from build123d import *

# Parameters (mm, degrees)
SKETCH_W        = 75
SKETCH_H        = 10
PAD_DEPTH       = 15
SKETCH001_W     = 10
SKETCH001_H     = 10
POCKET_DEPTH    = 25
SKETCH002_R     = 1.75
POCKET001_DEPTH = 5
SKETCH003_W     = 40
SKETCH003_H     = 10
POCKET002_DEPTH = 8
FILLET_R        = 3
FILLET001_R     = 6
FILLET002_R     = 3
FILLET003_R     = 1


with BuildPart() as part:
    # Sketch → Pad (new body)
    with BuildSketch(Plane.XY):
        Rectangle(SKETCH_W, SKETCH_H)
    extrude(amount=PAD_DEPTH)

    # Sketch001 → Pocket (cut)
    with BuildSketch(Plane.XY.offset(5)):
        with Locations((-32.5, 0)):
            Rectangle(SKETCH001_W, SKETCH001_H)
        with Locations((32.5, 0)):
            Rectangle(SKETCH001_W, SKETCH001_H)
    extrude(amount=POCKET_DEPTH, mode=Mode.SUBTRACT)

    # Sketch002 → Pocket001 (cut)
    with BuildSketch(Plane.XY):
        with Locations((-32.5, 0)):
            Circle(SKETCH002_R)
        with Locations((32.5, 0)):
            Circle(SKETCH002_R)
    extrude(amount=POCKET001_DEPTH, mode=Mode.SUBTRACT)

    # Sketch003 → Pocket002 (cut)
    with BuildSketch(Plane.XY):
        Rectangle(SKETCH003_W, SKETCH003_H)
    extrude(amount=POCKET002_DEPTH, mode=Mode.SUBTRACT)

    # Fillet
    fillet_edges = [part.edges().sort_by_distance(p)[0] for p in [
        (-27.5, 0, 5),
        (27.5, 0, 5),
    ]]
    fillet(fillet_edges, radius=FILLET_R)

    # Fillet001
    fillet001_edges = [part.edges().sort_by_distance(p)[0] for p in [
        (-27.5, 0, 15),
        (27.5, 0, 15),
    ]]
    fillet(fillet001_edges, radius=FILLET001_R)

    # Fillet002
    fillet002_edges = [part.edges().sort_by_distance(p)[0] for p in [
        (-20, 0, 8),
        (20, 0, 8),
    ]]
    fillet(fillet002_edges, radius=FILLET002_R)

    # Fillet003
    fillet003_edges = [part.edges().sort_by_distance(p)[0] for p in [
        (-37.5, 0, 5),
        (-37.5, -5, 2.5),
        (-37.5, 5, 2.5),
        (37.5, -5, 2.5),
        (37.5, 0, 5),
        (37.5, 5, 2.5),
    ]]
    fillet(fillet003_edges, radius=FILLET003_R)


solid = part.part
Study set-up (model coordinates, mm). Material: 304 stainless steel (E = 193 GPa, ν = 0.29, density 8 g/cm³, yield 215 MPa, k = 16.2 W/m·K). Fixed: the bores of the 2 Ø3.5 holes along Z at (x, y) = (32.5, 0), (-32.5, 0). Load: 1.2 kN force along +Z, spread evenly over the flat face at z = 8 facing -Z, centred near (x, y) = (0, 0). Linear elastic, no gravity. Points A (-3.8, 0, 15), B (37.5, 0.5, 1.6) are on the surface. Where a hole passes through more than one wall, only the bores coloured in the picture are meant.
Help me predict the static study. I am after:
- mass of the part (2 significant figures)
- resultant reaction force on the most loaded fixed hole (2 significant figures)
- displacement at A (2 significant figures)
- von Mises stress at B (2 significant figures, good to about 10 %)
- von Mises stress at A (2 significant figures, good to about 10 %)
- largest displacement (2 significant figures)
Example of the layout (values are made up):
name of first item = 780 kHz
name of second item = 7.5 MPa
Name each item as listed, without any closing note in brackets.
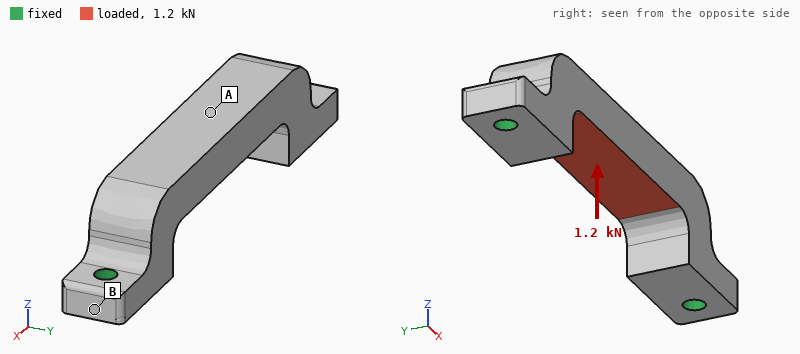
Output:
mass of the part = 47 g
resultant reaction force on the most loaded fixed hole = 1.1 kN
displacement at A = 12 µm
von Mises stress at B = 8.6 MPa
von Mises stress at A = 52 MPa
largest displacement = 13 µm
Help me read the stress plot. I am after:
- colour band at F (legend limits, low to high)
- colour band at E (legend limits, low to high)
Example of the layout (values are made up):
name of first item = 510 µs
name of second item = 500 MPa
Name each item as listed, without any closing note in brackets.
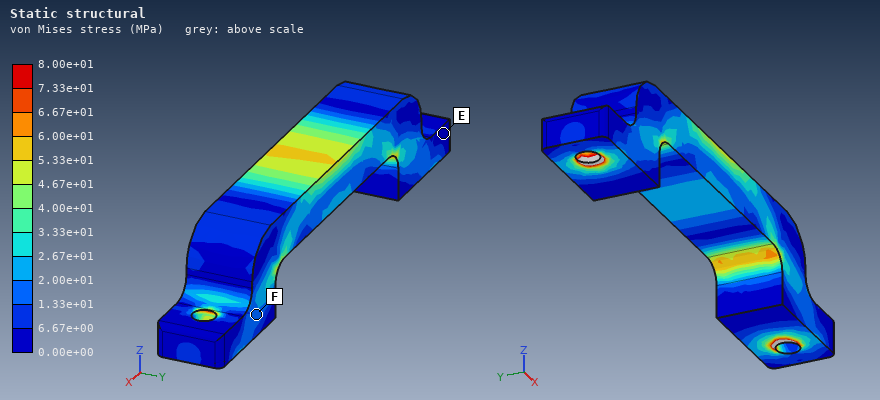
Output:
colour band at F = 1.33e+01 to 2.00e+01 MPa
colour band at E = 0.00e+00 to 6.67e+00 MPa
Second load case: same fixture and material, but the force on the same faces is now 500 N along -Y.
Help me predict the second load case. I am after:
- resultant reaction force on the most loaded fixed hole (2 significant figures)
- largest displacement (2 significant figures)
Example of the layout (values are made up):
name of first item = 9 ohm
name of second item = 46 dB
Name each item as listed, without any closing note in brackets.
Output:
resultant reaction force on the most loaded fixed hole = 250 N
largest displacement = 12 µm
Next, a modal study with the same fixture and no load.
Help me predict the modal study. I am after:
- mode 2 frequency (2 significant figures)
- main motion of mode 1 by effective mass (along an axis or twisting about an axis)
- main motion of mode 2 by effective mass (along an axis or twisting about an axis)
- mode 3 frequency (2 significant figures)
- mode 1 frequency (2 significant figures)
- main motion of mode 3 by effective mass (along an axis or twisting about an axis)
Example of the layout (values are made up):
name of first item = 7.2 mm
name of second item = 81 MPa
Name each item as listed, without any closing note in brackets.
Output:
mode 2 frequency = 11 kHz
main motion of mode 1 by effective mass = along Y
main motion of mode 2 by effective mass = along Z
mode 3 frequency = 13 kHz
mode 1 frequency = 6500 Hz
main motion of mode 3 by effective mass = along X
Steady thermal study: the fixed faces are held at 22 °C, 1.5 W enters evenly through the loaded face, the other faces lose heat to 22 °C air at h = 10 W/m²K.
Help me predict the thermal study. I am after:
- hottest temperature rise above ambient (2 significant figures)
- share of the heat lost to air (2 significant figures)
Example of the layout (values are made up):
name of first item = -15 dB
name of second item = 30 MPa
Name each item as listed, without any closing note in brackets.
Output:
hottest temperature rise above ambient = 16 K
share of the heat lost to air = 13 %
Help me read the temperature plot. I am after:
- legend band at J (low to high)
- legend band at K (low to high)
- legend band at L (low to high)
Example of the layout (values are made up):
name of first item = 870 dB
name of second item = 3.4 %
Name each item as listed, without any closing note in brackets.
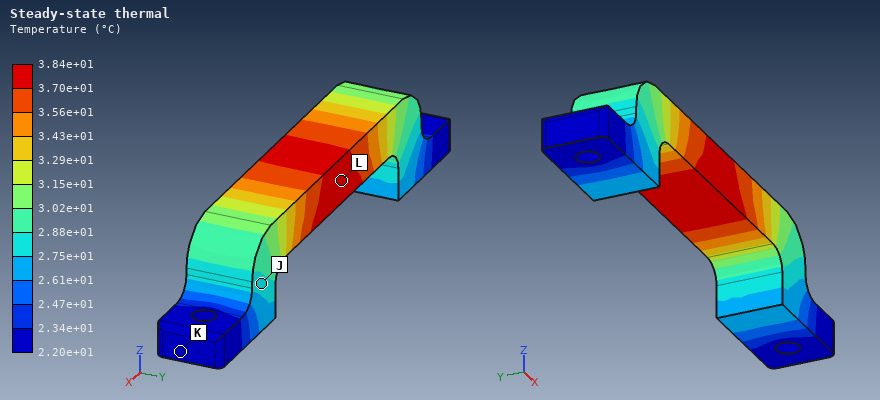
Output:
legend band at J = 2.75e+01 to 2.88e+01 °C
legend band at K = 2.20e+01 to 2.34e+01 °C
legend band at L = 3.70e+01 to 3.84e+01 °C
